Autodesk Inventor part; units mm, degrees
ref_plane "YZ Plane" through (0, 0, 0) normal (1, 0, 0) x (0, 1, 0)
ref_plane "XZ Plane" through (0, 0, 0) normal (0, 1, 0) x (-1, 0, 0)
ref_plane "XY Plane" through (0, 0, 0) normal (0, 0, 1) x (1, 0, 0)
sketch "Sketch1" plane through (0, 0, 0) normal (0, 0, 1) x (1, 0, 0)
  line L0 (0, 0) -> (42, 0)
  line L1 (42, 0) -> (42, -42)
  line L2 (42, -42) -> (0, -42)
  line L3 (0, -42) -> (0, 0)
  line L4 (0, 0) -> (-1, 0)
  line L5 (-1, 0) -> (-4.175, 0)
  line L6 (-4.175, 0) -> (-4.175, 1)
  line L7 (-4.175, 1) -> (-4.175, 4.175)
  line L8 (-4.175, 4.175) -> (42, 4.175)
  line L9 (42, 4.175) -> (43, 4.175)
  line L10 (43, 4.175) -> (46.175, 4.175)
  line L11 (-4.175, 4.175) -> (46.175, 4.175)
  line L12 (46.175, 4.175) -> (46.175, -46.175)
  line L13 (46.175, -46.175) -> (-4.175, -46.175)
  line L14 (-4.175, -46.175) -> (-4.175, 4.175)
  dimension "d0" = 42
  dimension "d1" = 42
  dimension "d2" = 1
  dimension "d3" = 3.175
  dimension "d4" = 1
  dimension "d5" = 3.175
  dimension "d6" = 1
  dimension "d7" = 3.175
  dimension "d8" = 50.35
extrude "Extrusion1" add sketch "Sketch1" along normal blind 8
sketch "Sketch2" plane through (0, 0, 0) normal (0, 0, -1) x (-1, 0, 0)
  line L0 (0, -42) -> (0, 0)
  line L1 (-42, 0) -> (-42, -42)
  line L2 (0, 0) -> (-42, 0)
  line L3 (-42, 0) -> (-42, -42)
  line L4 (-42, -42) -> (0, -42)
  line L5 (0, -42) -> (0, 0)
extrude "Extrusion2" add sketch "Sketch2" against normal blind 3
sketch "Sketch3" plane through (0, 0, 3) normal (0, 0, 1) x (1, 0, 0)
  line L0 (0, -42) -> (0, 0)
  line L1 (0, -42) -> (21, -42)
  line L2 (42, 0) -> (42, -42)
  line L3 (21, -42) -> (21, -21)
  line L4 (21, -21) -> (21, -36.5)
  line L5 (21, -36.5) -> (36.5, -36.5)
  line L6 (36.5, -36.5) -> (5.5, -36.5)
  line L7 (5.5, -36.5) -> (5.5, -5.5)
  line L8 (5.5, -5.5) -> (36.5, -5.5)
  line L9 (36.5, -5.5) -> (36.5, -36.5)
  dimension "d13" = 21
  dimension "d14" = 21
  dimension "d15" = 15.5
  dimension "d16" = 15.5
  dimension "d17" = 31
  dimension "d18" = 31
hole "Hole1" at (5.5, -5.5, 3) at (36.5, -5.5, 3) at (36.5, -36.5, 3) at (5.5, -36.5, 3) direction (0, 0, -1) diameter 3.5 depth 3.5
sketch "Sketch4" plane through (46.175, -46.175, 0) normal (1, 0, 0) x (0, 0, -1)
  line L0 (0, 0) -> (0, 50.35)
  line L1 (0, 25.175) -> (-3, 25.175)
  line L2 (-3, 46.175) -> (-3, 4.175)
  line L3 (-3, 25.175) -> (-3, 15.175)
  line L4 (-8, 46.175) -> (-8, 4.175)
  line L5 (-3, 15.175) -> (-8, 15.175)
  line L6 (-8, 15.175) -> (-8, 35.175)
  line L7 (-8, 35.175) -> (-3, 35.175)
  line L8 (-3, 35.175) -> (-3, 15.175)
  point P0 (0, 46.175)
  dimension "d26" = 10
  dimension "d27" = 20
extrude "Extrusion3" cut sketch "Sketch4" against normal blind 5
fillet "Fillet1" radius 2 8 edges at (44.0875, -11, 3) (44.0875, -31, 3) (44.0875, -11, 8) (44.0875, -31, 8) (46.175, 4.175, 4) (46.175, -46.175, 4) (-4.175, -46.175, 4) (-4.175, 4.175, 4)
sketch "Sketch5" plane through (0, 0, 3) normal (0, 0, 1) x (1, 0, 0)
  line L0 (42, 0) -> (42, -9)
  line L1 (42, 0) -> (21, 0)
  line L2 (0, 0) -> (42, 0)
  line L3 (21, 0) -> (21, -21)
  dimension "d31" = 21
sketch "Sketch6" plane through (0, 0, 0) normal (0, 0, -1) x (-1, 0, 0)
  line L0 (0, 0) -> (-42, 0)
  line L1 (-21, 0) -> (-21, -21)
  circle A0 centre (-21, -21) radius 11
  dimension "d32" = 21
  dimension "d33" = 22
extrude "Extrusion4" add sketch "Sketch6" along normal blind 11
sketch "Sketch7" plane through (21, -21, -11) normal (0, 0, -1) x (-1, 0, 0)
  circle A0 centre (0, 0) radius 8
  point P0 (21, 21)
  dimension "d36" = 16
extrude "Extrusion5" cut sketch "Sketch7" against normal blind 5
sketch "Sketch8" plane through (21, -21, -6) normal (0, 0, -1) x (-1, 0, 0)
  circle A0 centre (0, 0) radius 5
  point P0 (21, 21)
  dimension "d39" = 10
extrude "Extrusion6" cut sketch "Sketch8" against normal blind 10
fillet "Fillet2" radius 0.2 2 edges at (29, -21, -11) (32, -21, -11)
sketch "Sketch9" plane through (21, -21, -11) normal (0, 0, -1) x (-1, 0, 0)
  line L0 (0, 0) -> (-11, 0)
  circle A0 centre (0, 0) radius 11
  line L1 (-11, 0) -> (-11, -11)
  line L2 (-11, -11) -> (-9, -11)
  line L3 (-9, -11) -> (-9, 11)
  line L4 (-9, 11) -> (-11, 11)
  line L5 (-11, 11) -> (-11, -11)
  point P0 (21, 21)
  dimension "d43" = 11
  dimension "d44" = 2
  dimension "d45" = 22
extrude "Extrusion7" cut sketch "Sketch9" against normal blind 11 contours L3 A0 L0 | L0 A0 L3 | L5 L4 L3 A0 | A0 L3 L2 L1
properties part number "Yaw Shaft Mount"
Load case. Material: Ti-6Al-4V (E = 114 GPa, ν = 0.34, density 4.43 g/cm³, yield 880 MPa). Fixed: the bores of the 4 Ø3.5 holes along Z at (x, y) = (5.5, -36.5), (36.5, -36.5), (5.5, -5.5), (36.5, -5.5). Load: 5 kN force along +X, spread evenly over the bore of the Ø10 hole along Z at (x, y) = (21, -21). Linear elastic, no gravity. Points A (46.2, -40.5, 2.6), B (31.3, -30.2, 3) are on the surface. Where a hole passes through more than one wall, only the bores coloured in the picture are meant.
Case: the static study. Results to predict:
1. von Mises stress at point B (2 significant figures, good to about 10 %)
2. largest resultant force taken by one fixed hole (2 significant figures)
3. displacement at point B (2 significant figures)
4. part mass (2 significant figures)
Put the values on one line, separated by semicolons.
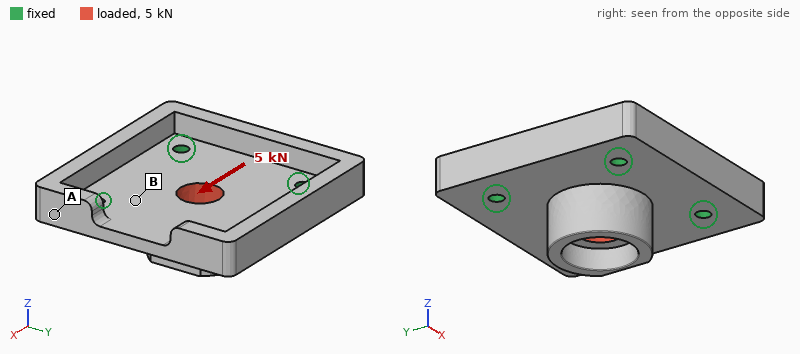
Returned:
27 MPa; 1.3 kN; 7.4 µm; 58 g
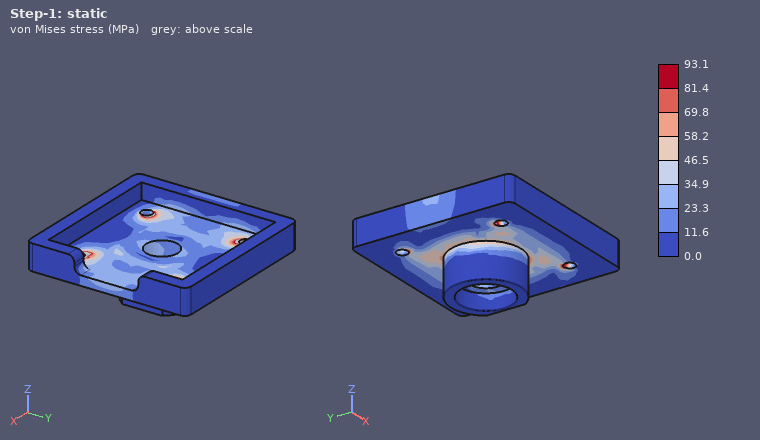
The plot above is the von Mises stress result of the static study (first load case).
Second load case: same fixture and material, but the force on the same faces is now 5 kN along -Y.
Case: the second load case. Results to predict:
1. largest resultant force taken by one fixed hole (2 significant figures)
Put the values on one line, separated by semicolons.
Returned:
1.3 kN
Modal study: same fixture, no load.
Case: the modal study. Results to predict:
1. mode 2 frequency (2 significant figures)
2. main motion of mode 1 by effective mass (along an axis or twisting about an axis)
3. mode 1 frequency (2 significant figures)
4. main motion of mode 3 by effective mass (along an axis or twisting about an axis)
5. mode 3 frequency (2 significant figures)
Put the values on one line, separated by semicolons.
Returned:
13 kHz; along Z; 11 kHz; twisting about X; 14 kHz
